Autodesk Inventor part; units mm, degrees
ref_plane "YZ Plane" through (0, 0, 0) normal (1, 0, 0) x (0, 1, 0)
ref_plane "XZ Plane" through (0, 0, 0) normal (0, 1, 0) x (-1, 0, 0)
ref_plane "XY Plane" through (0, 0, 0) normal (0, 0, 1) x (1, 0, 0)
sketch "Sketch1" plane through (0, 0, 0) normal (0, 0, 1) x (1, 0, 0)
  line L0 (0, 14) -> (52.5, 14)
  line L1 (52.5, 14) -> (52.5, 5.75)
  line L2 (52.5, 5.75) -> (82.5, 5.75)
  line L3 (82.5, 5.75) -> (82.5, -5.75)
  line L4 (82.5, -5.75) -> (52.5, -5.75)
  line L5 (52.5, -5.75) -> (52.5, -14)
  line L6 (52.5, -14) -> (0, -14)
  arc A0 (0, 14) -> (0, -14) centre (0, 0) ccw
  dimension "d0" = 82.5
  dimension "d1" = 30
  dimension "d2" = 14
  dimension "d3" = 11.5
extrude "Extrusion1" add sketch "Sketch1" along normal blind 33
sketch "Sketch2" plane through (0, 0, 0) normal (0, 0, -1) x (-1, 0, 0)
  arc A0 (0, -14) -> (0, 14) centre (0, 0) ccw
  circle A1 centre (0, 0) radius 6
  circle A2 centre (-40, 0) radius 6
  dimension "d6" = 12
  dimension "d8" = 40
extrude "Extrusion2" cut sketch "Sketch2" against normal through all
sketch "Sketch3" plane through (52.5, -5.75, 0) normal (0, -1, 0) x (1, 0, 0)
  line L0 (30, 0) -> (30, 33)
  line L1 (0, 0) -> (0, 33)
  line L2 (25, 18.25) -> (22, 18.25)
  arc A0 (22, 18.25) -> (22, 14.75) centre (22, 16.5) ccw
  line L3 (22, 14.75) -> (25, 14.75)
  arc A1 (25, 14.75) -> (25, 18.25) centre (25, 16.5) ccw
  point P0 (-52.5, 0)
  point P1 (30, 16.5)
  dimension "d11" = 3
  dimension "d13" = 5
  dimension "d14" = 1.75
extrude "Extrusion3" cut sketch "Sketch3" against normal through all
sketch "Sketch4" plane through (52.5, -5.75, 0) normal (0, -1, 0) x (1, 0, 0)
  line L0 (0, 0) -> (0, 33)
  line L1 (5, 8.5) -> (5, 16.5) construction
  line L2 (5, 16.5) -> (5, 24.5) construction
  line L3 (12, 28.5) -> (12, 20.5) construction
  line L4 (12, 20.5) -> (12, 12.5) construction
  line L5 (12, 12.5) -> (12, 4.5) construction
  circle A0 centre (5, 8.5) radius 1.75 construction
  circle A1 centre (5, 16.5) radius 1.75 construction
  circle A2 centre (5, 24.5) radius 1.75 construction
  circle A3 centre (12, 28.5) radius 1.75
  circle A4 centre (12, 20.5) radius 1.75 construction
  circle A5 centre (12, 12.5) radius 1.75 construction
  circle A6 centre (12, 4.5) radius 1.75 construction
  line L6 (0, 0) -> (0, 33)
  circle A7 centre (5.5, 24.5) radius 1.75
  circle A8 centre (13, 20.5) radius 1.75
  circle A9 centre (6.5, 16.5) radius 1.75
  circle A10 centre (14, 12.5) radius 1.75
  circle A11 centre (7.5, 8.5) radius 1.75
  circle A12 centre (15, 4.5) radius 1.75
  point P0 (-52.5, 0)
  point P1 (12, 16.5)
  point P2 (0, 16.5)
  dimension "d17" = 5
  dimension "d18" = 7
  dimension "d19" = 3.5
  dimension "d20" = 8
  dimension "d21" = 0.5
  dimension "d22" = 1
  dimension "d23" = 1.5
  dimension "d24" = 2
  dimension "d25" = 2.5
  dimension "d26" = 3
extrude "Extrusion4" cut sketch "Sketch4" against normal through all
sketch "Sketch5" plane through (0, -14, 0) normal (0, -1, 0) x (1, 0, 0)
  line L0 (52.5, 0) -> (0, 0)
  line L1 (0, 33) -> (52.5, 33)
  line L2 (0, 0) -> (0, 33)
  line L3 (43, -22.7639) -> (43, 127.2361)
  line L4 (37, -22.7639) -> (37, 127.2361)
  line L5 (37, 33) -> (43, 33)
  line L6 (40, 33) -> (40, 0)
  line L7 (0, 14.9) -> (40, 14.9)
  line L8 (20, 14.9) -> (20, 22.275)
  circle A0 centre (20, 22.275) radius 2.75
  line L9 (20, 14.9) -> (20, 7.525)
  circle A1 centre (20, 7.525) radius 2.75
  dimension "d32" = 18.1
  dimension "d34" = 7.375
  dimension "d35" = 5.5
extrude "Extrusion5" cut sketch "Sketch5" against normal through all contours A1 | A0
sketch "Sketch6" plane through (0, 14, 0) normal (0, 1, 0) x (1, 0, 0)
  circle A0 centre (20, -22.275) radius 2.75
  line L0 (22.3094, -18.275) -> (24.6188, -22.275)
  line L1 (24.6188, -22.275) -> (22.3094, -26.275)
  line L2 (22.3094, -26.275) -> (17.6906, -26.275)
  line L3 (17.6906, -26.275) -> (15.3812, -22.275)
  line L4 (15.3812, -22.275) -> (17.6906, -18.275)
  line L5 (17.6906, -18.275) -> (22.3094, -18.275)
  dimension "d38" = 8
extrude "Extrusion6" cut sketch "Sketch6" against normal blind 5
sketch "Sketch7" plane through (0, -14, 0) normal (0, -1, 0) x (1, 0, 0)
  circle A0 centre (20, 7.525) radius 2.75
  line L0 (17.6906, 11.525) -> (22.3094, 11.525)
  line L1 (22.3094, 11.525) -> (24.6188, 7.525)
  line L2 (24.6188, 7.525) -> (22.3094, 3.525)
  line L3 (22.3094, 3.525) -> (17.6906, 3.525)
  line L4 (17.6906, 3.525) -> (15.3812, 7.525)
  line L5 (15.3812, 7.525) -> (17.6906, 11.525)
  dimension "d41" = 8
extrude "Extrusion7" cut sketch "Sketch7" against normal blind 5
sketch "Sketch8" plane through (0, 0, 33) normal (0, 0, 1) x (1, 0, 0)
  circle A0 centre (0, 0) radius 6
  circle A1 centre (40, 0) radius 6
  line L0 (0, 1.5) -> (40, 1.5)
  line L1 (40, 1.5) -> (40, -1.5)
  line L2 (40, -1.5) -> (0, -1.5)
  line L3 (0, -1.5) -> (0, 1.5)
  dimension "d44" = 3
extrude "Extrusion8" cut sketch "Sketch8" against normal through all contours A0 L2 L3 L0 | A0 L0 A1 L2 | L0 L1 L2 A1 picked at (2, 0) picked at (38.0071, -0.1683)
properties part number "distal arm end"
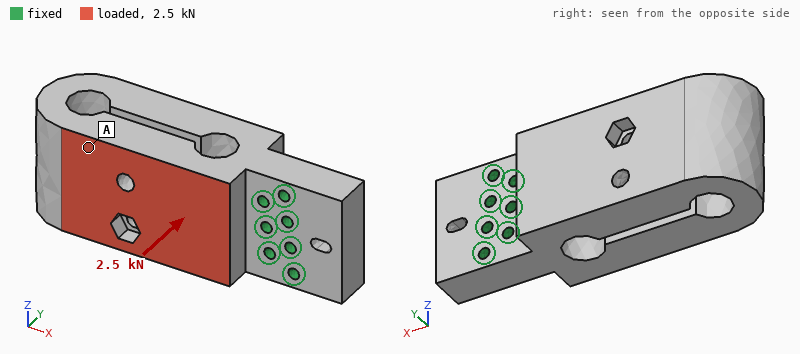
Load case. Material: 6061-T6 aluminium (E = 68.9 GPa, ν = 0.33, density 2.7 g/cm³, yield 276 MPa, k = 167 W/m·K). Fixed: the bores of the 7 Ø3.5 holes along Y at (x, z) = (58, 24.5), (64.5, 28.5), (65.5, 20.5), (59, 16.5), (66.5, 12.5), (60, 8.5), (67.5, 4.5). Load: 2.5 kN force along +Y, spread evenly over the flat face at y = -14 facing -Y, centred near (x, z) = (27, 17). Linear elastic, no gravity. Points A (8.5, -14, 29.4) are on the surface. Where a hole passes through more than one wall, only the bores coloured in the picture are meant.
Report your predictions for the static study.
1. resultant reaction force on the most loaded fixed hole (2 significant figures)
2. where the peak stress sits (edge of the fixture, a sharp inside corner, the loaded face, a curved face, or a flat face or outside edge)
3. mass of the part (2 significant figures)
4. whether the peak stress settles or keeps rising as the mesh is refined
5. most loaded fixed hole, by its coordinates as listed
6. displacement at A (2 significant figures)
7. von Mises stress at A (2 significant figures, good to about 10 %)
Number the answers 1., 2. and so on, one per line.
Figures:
1. 1.5 kN
2. edge of the fixture
3. 150 g
4. keeps rising
5. (58, 24.5)
6. 0.20 mm
7. 15 MPa
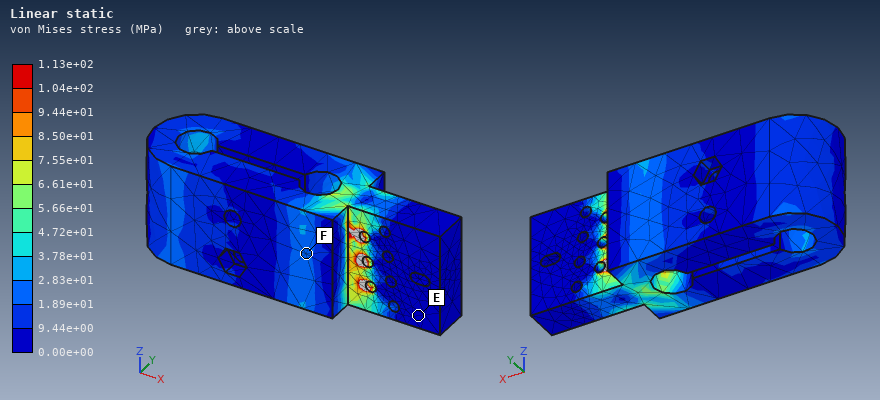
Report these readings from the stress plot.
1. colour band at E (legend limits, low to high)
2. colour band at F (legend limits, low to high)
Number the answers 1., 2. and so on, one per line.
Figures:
1. 0.00e+00 to 9.44e+00 MPa
2. 1.89e+01 to 2.83e+01 MPa
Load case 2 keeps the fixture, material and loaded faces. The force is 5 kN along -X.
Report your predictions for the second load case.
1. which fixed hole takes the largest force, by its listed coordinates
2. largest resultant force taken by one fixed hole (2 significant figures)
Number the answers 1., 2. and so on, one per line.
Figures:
1. (58, 24.5)
2. 1.6 kN
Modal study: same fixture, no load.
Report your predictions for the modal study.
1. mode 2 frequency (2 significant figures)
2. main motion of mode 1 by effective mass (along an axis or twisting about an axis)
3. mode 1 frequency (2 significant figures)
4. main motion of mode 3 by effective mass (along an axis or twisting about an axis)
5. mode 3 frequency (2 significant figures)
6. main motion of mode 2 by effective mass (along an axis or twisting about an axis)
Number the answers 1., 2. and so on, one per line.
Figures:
1. 3100 Hz
2. along Y
3. 1500 Hz
4. twisting about X
5. 6200 Hz
6. along Z
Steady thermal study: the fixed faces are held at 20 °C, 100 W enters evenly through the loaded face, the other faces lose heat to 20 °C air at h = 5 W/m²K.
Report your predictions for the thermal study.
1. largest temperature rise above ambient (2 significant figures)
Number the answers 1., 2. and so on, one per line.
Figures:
1. 47 K
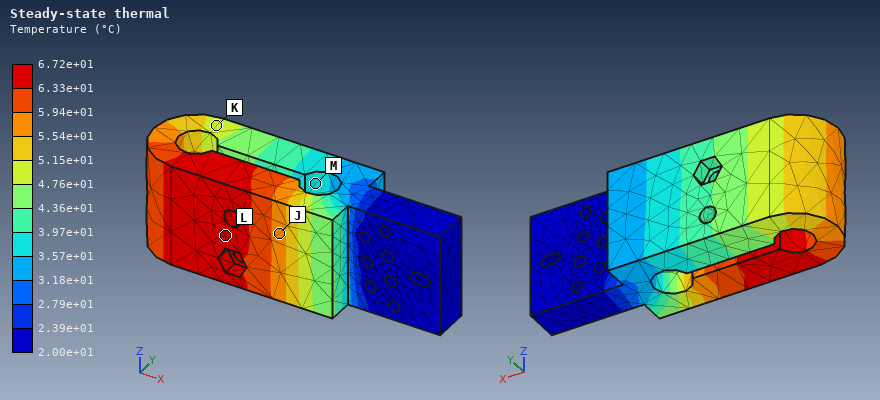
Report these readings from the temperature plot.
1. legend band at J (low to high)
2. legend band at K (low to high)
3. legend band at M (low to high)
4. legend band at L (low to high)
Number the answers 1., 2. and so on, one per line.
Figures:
1. 5.54e+01 to 5.94e+01 °C
2. 4.76e+01 to 5.15e+01 °C
3. 3.57e+01 to 3.97e+01 °C
4. 6.33e+01 to 6.72e+01 °C
